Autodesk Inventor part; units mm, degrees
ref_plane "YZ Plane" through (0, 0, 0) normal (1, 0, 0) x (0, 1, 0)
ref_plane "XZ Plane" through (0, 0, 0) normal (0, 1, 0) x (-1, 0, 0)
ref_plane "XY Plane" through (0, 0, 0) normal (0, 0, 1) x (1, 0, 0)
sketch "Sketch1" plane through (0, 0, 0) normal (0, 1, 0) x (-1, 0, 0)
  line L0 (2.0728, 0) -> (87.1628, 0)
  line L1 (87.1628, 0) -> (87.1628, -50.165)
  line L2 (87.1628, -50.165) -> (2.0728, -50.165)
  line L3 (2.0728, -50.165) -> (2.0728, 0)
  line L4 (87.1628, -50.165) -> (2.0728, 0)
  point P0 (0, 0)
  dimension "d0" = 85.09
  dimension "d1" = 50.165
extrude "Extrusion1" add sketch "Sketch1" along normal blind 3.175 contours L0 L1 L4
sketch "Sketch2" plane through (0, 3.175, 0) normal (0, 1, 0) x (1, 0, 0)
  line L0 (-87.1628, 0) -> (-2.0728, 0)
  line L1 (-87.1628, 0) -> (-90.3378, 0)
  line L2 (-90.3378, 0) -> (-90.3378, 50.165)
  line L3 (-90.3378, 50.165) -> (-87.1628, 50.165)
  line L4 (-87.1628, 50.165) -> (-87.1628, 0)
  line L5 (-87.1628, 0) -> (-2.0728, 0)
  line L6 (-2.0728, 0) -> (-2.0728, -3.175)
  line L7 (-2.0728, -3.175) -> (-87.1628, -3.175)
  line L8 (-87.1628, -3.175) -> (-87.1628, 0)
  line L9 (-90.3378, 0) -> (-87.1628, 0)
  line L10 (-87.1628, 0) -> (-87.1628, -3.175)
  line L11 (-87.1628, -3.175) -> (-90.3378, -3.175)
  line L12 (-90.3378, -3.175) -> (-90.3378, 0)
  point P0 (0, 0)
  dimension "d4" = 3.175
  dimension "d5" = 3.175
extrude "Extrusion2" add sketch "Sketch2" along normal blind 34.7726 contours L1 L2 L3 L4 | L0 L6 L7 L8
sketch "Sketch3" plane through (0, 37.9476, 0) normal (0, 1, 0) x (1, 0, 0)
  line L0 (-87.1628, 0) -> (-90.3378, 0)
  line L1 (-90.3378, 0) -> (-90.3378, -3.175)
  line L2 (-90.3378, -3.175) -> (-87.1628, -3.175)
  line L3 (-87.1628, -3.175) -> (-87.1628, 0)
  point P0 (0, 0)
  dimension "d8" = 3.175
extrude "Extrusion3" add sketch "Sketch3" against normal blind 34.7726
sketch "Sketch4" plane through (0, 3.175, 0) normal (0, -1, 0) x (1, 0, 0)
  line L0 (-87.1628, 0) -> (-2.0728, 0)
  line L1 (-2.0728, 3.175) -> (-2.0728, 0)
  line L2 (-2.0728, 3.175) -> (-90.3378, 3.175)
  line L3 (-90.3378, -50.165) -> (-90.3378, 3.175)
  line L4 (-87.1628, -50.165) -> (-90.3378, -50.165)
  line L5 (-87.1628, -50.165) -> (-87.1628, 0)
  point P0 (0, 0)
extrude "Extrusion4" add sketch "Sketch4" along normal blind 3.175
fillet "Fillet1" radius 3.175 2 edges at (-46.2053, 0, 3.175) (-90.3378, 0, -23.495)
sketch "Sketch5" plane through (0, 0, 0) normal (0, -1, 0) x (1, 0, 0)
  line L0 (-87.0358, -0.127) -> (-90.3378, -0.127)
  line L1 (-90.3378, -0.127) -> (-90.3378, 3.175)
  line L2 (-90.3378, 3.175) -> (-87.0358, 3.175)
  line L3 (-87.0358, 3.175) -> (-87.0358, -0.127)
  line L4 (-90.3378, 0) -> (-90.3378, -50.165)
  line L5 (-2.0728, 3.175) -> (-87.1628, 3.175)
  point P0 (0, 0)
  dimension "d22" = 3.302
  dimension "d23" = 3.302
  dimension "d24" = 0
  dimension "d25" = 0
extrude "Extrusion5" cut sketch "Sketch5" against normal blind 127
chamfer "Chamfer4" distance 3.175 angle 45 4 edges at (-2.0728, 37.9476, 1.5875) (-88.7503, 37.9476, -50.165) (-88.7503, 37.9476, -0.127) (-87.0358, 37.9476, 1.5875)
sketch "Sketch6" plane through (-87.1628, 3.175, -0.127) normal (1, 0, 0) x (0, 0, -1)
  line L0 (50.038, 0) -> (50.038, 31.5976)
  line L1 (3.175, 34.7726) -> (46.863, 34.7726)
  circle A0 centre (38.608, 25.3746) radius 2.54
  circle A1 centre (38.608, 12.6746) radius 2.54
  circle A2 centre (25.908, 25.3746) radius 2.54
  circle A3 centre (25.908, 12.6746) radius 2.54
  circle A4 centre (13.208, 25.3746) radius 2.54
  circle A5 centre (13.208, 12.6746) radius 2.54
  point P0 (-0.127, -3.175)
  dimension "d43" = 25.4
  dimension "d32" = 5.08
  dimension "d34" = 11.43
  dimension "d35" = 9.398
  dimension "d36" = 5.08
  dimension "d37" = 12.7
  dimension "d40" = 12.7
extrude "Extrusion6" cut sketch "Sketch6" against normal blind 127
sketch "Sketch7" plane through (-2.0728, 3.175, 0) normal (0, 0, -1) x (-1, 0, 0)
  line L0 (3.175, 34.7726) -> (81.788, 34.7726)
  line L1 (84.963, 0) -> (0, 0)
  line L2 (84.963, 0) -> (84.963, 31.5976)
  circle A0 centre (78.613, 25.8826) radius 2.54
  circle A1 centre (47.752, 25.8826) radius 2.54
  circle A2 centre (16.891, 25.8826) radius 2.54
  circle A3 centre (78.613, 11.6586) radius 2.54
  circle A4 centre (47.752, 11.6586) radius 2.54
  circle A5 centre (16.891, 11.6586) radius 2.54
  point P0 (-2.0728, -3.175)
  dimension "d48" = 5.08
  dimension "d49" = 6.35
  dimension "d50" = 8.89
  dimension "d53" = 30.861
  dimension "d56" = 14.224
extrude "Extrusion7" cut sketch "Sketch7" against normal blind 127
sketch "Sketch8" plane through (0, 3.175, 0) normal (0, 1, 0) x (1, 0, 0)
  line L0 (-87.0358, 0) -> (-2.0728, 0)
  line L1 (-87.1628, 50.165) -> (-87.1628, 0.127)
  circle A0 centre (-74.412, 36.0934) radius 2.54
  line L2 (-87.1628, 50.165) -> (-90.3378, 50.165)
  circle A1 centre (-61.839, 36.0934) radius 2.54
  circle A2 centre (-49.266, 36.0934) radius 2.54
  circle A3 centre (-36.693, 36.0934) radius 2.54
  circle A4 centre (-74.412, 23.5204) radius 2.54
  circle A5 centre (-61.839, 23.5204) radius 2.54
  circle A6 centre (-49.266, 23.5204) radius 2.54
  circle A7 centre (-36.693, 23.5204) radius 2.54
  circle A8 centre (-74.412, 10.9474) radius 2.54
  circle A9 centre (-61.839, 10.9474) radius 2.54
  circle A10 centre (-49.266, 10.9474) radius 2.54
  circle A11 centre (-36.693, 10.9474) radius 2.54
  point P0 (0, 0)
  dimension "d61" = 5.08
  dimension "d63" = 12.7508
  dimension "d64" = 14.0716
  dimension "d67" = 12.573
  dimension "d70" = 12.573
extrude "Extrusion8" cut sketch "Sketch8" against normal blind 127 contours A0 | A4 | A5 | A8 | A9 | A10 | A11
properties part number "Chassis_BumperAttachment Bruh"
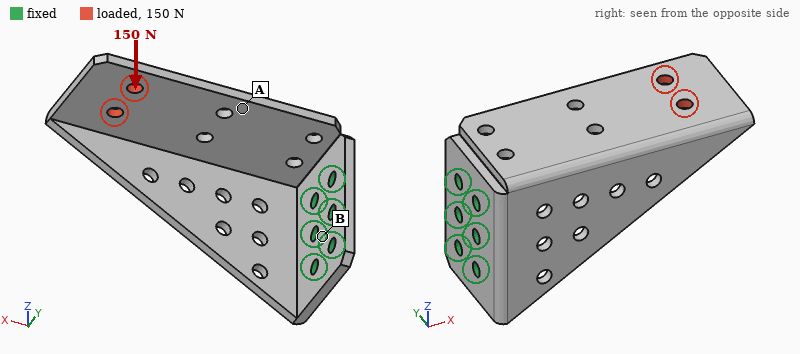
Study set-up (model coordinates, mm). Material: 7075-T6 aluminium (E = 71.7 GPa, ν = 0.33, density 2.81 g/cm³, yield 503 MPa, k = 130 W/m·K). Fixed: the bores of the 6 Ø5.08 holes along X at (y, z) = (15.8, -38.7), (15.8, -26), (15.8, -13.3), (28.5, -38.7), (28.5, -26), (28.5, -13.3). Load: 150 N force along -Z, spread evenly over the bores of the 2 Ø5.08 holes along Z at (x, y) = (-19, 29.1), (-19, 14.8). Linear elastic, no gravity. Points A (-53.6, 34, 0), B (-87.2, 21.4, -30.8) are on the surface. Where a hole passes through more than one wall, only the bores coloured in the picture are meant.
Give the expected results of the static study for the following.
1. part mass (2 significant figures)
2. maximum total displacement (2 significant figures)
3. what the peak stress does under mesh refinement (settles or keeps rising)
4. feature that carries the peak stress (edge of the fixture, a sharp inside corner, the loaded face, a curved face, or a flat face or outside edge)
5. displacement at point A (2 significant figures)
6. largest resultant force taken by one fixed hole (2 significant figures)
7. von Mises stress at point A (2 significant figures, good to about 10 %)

60 g
1.1 mm
keeps rising
a sharp inside corner
0.56 mm
390 N
22 MPa
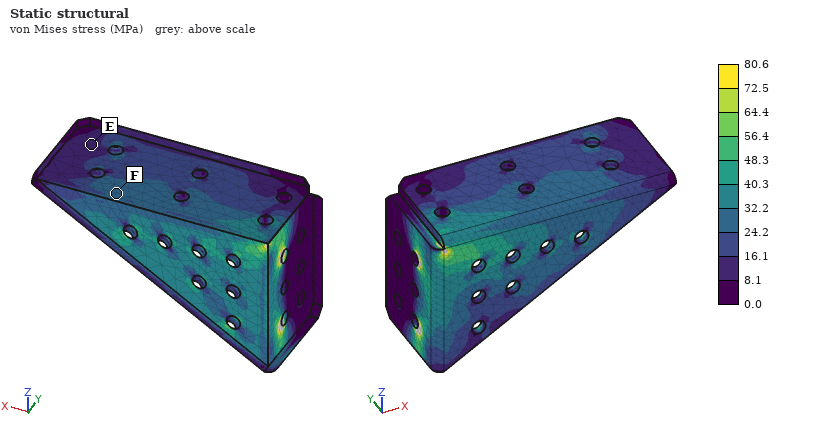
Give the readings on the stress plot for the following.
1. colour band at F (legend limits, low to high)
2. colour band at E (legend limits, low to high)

24.2 to 32.2 MPa
8.1 to 16.1 MPa
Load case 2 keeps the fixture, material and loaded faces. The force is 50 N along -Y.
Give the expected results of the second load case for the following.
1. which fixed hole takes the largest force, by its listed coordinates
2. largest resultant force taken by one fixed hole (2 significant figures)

(15.8, -13.3)
60 N
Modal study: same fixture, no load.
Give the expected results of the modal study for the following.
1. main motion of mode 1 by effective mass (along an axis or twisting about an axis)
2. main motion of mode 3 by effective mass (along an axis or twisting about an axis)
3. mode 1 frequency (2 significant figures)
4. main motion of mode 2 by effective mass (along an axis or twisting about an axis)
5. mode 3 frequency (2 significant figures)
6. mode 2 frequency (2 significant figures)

along Y
along X
280 Hz
along Z
1400 Hz
670 Hz
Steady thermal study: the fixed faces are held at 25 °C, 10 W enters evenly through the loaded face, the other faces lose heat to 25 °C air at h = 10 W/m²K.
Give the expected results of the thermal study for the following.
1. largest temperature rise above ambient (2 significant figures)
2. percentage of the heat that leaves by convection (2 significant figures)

42 K
27 %
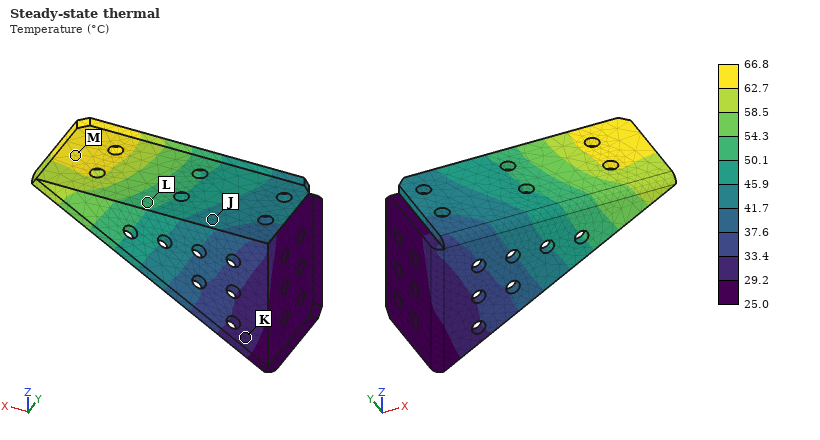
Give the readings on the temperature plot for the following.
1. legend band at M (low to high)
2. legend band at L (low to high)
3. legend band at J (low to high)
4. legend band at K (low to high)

62.7 to 66.8 °C
50.1 to 54.3 °C
41.7 to 45.9 °C
29.2 to 33.4 °C
